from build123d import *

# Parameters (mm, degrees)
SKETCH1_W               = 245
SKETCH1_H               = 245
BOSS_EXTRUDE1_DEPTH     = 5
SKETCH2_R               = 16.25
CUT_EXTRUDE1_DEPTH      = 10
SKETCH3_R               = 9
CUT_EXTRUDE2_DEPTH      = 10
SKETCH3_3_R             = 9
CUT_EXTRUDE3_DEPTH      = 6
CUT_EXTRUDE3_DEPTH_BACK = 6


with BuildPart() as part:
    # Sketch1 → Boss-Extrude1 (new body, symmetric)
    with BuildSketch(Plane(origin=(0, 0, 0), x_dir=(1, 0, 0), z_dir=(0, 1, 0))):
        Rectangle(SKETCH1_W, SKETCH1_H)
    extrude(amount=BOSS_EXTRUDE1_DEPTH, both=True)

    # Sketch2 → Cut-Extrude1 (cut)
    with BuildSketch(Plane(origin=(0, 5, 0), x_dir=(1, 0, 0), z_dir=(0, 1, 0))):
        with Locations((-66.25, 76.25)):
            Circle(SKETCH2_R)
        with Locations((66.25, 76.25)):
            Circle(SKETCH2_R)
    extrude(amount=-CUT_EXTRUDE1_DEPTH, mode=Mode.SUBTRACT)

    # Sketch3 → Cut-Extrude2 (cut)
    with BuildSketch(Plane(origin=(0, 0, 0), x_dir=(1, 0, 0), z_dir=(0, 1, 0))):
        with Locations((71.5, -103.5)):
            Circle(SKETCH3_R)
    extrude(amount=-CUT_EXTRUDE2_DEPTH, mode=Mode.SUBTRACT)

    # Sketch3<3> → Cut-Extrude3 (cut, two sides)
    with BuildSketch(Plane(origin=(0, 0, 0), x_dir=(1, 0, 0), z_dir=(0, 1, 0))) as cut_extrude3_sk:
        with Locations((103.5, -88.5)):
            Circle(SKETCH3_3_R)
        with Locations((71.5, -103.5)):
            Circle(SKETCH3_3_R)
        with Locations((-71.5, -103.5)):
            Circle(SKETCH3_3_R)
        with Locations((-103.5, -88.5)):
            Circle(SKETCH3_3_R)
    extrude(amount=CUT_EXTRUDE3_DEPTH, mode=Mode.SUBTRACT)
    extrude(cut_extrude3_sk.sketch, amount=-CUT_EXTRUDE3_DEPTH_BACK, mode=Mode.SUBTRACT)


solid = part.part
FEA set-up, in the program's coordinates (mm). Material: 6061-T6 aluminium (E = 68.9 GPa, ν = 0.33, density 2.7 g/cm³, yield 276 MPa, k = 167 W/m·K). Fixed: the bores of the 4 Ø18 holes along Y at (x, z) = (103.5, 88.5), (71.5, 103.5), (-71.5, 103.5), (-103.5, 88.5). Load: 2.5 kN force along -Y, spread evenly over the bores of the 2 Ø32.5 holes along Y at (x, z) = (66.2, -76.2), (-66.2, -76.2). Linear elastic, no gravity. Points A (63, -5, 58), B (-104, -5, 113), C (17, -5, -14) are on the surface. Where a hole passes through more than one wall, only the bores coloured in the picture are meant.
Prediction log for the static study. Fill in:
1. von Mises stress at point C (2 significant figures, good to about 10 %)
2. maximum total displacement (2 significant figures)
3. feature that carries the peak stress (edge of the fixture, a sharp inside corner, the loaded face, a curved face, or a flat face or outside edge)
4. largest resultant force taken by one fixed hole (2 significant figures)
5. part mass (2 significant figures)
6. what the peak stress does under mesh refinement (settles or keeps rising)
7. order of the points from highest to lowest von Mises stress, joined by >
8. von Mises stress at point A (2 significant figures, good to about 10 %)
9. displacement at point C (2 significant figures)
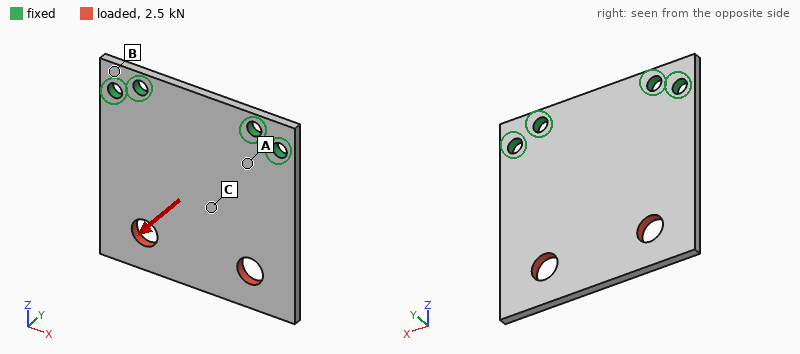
37 MPa
4.2 mm
edge of the fixture
1.6 kN
1.5 kg
keeps rising
A > C > B
74 MPa
1.5 mm
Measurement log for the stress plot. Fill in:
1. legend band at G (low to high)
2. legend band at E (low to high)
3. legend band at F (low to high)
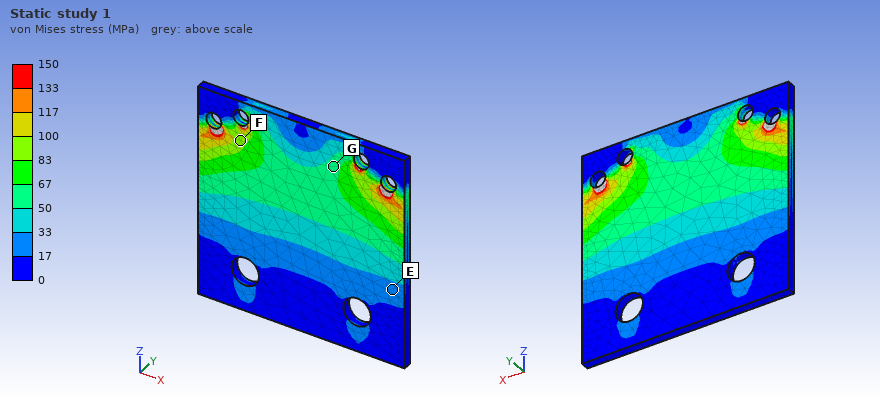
50 to 67 MPa
17 to 33 MPa
83 to 100 MPa
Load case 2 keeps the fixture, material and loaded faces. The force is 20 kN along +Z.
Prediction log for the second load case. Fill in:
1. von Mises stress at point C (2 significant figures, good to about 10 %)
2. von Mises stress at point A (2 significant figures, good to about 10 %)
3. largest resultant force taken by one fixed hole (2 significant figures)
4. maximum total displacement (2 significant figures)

6.3 MPa
10 MPa
5.3 kN
31 µm
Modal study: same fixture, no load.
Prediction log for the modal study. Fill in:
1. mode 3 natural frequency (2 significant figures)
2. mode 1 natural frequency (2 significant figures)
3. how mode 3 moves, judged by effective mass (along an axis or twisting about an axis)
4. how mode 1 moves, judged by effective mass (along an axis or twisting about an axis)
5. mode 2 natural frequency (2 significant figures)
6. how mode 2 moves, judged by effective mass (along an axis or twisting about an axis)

1100 Hz
180 Hz
along Y
along Y
420 Hz
twisting about Z
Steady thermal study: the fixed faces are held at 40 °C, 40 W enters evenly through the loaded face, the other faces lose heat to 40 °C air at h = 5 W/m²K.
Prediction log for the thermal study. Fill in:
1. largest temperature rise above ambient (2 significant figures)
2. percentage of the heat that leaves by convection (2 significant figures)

18 K
14 %
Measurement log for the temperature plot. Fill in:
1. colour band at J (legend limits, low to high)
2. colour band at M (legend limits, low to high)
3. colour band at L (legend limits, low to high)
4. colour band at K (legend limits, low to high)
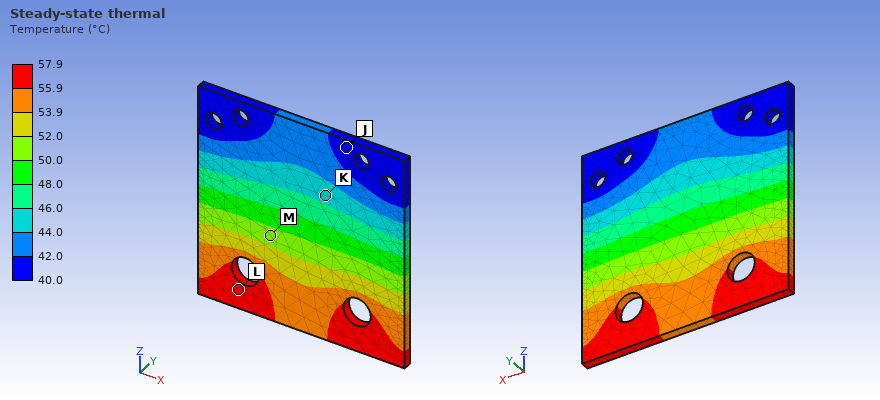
40.0 to 42.0 °C
50.0 to 52.0 °C
55.9 to 57.9 °C
44.0 to 46.0 °C
